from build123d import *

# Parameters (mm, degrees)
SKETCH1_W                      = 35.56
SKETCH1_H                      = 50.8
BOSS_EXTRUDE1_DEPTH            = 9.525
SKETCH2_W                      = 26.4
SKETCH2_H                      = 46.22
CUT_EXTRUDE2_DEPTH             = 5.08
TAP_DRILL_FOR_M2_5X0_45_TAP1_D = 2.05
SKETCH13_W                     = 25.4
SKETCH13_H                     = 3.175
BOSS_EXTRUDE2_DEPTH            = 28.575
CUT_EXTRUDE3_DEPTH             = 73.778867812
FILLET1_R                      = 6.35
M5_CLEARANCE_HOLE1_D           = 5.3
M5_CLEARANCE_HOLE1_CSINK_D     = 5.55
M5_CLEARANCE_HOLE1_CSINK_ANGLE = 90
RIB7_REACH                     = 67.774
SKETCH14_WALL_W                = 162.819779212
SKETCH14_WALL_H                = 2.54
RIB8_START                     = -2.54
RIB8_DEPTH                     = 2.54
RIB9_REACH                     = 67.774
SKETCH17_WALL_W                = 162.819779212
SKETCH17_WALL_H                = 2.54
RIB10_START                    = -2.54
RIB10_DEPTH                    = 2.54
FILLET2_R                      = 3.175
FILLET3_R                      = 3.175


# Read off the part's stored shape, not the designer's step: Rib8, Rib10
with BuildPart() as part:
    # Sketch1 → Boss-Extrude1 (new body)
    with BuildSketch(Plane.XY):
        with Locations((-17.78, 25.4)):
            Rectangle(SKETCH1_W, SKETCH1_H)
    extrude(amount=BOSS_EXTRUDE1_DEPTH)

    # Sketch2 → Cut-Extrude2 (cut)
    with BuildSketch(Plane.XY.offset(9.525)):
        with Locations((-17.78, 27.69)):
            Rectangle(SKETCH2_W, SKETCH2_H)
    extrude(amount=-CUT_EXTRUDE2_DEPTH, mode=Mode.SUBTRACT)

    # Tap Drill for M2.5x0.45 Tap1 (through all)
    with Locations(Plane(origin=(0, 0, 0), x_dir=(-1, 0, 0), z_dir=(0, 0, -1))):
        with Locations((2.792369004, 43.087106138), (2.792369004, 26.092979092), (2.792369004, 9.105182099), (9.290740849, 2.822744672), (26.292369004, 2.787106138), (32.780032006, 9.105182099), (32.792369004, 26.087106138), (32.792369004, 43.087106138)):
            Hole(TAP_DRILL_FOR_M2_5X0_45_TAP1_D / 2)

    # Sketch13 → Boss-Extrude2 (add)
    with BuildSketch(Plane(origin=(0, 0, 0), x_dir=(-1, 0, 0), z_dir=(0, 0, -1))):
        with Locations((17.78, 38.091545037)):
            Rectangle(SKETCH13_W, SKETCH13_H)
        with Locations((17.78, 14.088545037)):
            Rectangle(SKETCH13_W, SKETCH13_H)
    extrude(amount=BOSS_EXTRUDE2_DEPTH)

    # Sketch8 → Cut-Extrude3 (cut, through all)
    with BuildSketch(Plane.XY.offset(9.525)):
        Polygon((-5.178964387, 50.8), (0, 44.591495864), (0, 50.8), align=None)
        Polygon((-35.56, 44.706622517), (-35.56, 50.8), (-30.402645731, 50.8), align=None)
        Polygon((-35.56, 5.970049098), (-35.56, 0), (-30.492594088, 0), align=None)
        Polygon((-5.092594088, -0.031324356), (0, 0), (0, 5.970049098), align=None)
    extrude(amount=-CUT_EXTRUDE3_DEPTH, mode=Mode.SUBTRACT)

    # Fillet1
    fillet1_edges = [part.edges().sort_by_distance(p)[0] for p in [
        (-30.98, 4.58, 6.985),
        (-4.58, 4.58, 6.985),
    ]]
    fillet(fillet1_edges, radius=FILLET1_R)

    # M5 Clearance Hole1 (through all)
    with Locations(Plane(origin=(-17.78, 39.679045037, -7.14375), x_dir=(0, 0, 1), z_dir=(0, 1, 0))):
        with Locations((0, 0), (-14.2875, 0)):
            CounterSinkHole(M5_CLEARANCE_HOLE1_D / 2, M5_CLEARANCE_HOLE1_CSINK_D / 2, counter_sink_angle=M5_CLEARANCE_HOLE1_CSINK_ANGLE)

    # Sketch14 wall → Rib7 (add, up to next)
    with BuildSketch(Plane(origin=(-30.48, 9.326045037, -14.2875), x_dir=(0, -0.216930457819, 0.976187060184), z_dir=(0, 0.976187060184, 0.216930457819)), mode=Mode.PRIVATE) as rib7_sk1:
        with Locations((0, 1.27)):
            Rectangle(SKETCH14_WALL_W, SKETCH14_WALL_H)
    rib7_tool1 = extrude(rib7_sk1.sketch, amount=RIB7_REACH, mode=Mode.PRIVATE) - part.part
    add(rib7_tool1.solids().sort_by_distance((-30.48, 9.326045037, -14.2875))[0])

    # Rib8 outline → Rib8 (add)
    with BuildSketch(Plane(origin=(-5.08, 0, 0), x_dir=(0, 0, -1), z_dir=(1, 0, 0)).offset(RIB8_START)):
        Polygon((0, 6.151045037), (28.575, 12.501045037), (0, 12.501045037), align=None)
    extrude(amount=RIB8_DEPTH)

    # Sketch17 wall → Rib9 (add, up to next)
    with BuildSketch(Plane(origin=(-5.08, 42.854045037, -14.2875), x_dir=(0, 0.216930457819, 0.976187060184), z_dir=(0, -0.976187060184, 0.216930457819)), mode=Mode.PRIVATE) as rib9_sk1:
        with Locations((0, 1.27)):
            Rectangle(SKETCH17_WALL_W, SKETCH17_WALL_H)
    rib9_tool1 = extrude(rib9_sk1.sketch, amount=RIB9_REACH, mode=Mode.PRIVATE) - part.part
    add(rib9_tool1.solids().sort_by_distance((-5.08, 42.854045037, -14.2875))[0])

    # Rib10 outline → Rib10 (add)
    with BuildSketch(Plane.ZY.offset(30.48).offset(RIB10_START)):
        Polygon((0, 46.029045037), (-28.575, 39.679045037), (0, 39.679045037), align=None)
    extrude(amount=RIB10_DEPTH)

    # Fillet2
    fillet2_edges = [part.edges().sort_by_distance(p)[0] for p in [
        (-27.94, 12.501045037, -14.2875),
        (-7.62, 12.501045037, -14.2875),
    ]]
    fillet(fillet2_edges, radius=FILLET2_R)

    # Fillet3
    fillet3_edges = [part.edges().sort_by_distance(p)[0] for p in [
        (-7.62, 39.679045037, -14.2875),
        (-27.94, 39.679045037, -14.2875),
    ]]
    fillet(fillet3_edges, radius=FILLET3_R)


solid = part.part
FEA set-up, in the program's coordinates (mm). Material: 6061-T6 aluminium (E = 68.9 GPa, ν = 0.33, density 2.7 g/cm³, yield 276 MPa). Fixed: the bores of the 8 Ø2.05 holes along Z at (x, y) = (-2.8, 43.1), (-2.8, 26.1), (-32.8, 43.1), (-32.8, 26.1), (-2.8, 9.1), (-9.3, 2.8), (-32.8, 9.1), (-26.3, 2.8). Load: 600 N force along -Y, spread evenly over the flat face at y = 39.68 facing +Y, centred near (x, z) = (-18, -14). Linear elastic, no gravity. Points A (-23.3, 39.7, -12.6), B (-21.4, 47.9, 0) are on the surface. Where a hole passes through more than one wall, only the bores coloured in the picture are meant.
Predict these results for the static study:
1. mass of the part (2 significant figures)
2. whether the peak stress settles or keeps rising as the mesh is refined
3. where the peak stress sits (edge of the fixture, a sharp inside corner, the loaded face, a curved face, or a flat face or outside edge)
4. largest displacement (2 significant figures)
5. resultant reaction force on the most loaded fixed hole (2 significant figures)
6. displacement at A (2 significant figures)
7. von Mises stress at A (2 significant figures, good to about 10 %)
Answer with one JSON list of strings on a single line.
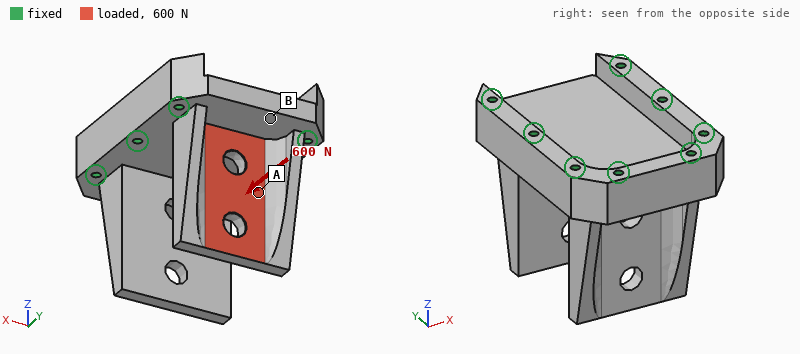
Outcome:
["42 g", "keeps rising", "edge of the fixture", "0.12 mm", "290 N", "0.037 mm", "19 MPa"]
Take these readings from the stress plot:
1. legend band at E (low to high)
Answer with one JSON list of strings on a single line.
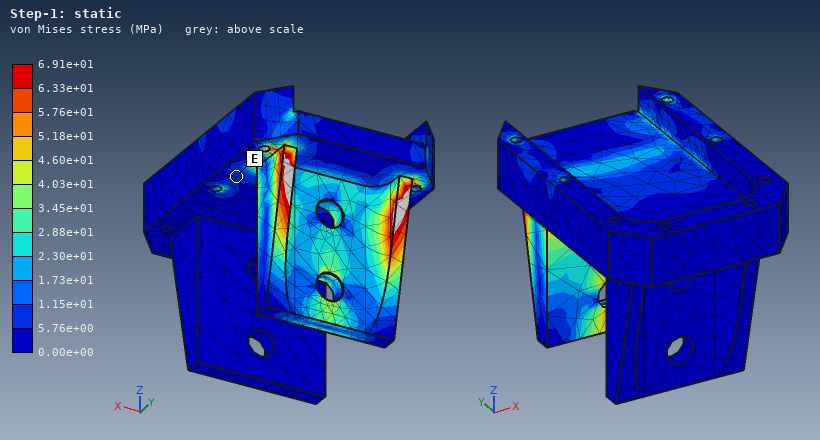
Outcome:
["5.76e+00 to 1.15e+01 MPa"]
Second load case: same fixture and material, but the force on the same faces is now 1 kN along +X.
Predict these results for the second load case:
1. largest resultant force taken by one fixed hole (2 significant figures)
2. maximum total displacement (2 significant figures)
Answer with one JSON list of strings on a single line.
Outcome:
["580 N", "41 µm"]
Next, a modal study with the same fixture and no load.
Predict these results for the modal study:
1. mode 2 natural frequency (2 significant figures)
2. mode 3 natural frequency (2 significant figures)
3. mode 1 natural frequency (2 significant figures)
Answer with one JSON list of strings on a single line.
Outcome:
["6000 Hz", "10 kHz", "5900 Hz"]
